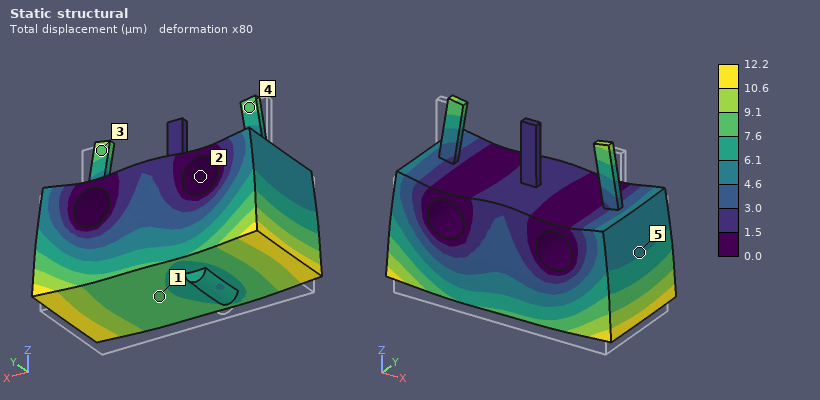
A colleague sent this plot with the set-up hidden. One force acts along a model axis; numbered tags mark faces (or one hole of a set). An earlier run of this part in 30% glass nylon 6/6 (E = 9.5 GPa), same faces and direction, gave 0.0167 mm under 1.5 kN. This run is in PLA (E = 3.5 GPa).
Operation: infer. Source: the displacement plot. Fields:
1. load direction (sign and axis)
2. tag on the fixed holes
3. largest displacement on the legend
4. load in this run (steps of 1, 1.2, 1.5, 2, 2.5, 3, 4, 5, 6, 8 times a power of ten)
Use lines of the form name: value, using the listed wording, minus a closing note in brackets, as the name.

load direction: +Z
tag on the fixed holes: 2
largest displacement on the legend: 12.2 µm
load in this run: 400 N
